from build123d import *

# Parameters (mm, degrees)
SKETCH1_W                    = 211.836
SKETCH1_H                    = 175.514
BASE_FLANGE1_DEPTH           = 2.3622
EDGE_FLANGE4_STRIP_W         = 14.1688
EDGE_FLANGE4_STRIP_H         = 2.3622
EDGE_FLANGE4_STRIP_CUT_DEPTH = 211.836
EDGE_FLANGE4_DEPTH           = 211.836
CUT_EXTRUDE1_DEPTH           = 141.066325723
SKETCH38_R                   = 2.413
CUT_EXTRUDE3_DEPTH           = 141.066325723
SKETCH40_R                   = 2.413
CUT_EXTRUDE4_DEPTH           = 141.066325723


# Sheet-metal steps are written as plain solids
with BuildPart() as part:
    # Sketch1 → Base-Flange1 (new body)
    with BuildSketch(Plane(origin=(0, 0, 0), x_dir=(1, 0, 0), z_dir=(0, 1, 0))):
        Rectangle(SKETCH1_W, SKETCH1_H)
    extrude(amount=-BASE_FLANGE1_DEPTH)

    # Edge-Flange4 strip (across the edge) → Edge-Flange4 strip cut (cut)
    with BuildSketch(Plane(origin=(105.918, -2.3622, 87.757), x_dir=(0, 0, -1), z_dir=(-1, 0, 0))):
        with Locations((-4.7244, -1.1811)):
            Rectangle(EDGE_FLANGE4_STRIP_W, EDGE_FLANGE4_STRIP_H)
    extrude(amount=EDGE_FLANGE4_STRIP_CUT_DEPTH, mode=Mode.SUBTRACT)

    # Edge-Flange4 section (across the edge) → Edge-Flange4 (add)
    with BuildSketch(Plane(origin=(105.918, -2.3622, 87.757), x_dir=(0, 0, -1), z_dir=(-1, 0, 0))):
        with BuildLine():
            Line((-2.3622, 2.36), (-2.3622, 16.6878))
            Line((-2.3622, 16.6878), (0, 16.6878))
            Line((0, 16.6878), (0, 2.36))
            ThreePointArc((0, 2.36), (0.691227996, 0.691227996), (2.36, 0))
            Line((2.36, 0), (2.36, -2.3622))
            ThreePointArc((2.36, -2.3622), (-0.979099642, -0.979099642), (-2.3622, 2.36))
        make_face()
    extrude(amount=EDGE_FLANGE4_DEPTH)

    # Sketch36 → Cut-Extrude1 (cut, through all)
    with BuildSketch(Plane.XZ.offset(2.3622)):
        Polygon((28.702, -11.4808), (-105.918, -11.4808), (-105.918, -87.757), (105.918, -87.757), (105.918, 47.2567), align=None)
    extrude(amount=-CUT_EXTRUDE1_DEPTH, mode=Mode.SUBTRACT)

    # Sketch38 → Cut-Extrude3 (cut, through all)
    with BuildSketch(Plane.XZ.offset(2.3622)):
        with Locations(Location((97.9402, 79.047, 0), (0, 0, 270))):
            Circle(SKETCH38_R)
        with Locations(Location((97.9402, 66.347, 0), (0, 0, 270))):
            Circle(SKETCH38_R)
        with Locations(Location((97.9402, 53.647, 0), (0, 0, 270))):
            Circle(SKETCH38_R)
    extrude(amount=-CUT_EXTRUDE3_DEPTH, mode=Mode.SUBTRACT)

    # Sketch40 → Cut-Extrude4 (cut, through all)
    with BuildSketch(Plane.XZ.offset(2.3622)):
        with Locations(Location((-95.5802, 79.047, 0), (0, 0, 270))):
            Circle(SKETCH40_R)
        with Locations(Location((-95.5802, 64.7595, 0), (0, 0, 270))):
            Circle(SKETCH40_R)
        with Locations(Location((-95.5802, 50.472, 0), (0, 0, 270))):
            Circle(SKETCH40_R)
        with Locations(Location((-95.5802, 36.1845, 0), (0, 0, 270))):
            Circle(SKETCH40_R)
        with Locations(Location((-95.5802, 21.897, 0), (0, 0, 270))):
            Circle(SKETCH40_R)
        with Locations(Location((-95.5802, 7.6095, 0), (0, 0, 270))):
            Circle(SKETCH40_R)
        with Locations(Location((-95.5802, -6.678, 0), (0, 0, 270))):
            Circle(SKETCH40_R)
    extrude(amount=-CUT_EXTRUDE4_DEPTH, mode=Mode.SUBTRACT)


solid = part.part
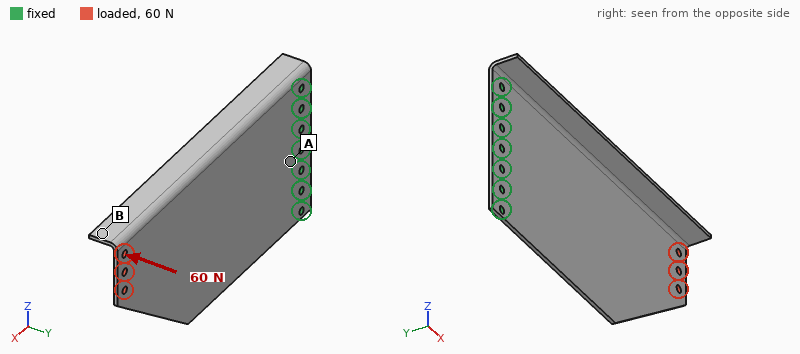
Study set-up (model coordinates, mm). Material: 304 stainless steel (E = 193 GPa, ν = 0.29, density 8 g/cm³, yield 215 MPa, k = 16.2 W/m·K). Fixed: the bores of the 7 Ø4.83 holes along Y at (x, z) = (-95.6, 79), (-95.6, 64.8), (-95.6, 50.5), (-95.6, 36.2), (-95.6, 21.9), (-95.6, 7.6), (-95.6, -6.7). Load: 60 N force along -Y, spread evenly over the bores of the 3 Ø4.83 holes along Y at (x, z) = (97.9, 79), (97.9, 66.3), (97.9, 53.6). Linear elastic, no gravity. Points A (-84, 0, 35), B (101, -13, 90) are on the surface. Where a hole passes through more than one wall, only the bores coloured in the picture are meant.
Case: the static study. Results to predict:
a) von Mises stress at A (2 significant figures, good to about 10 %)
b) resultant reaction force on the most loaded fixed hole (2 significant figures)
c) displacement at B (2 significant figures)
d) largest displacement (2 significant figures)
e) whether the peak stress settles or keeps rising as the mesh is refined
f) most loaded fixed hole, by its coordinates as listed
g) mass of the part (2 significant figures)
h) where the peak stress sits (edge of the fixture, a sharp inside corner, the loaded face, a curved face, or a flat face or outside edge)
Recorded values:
41 MPa
260 N
1.4 mm
1.5 mm
keeps rising
(-95.6, 79)
420 g
edge of the fixture
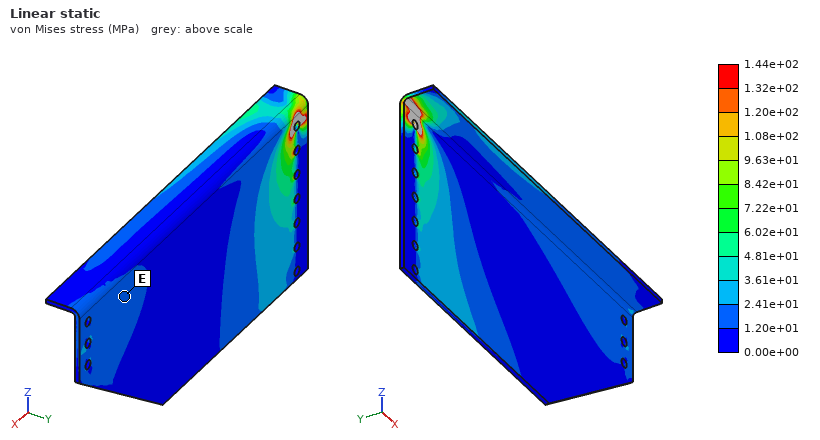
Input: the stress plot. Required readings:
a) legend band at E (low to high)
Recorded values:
1.20e+01 to 2.41e+01 MPa
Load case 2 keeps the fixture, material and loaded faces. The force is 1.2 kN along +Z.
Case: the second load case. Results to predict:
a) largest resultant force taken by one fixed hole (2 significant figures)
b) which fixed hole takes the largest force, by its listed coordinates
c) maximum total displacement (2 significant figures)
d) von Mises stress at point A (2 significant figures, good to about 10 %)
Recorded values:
2.2 kN
(-95.6, 79)
0.26 mm
10 MPa
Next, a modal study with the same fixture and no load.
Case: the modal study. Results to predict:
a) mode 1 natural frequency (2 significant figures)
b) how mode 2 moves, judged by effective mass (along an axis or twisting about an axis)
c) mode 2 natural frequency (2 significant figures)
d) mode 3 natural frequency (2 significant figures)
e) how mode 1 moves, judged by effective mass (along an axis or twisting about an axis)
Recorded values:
100 Hz
twisting about X
240 Hz
590 Hz
along Y
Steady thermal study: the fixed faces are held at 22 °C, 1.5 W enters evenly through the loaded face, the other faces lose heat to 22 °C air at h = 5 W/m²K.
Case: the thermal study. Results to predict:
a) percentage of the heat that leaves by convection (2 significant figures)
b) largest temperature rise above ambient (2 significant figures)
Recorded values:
92 %
33 K
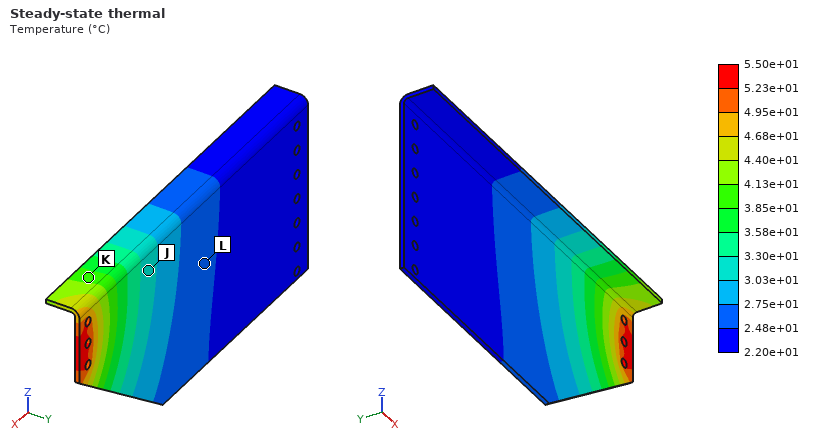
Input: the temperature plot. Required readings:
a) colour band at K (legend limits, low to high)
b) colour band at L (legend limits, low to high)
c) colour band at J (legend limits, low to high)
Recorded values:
3.85e+01 to 4.13e+01 °C
2.48e+01 to 2.75e+01 °C
3.03e+01 to 3.30e+01 °C
